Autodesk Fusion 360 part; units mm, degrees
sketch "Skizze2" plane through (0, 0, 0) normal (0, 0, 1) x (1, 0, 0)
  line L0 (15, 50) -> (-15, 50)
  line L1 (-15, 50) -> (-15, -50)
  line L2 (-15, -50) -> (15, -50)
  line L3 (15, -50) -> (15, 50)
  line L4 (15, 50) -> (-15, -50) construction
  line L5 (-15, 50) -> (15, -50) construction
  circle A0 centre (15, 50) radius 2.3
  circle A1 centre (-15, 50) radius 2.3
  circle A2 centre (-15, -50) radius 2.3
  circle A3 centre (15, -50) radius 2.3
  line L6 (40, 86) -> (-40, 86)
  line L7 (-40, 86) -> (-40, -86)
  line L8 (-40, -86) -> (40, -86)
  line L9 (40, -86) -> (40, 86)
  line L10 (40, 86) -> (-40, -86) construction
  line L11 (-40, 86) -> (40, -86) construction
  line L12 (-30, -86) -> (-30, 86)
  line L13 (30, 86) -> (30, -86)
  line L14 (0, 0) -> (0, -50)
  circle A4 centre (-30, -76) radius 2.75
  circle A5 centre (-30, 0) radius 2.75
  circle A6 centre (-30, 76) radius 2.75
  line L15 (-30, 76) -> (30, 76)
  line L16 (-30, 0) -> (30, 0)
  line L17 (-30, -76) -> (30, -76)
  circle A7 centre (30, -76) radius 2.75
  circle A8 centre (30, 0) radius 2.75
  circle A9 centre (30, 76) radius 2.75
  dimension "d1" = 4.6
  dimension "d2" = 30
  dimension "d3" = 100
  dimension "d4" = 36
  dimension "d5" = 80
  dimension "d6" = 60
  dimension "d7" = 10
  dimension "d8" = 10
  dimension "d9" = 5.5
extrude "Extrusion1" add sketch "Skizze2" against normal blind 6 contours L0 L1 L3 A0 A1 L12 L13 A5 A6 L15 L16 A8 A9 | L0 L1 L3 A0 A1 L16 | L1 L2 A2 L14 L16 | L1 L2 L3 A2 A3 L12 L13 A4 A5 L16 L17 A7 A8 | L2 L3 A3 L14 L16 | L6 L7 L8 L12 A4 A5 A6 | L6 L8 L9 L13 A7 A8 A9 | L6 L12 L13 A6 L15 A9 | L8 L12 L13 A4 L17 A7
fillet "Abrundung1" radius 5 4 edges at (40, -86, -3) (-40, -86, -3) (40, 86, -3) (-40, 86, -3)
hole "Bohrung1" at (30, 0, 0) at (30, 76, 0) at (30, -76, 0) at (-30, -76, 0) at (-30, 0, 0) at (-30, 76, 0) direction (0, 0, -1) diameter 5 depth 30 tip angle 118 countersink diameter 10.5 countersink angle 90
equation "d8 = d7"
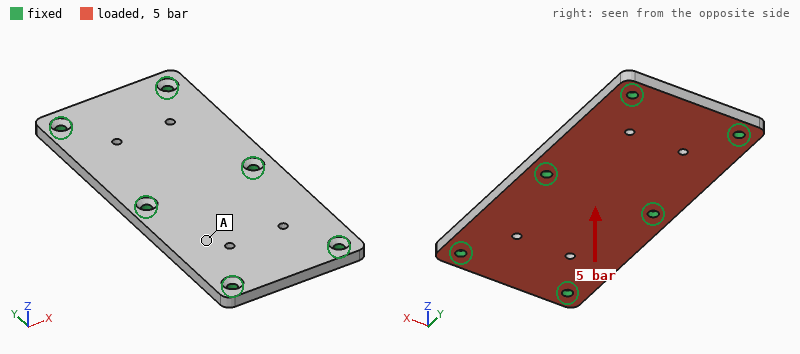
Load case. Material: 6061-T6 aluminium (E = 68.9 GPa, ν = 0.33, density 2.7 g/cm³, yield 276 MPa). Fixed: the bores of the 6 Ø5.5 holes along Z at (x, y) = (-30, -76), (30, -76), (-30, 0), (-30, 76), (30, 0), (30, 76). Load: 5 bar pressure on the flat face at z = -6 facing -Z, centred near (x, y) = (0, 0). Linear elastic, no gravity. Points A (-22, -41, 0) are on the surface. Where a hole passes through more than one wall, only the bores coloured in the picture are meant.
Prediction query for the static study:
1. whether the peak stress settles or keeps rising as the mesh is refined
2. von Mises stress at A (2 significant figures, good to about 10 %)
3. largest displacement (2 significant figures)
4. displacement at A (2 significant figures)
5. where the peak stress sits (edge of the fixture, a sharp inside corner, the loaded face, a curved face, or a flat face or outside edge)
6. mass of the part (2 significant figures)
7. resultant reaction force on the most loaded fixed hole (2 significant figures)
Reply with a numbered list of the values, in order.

1. keeps rising
2. 23 MPa
3. 68 µm
4. 57 µm
5. edge of the fixture
6. 220 g
7. 1.7 kN
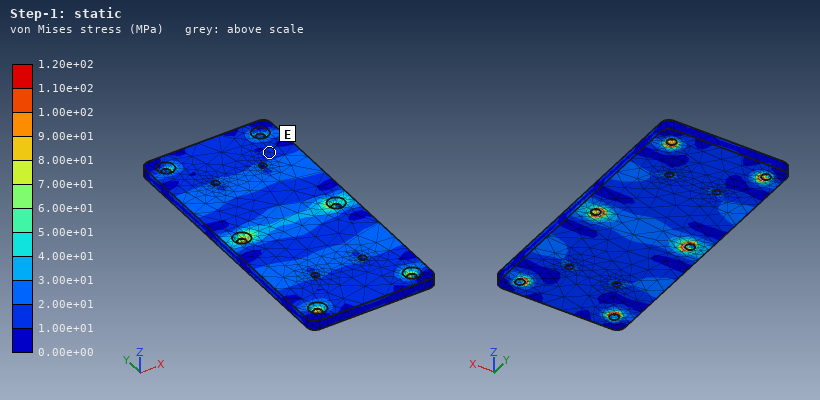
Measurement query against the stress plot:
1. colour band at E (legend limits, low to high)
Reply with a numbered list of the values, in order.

1. 1.00e+01 to 2.00e+01 MPa
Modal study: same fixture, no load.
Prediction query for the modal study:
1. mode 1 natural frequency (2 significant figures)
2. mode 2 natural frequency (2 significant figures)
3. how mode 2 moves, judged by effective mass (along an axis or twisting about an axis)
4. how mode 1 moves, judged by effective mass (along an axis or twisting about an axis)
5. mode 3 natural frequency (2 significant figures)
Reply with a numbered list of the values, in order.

1. 3800 Hz
2. 4000 Hz
3. along Z
4. twisting about X
5. 5400 Hz
